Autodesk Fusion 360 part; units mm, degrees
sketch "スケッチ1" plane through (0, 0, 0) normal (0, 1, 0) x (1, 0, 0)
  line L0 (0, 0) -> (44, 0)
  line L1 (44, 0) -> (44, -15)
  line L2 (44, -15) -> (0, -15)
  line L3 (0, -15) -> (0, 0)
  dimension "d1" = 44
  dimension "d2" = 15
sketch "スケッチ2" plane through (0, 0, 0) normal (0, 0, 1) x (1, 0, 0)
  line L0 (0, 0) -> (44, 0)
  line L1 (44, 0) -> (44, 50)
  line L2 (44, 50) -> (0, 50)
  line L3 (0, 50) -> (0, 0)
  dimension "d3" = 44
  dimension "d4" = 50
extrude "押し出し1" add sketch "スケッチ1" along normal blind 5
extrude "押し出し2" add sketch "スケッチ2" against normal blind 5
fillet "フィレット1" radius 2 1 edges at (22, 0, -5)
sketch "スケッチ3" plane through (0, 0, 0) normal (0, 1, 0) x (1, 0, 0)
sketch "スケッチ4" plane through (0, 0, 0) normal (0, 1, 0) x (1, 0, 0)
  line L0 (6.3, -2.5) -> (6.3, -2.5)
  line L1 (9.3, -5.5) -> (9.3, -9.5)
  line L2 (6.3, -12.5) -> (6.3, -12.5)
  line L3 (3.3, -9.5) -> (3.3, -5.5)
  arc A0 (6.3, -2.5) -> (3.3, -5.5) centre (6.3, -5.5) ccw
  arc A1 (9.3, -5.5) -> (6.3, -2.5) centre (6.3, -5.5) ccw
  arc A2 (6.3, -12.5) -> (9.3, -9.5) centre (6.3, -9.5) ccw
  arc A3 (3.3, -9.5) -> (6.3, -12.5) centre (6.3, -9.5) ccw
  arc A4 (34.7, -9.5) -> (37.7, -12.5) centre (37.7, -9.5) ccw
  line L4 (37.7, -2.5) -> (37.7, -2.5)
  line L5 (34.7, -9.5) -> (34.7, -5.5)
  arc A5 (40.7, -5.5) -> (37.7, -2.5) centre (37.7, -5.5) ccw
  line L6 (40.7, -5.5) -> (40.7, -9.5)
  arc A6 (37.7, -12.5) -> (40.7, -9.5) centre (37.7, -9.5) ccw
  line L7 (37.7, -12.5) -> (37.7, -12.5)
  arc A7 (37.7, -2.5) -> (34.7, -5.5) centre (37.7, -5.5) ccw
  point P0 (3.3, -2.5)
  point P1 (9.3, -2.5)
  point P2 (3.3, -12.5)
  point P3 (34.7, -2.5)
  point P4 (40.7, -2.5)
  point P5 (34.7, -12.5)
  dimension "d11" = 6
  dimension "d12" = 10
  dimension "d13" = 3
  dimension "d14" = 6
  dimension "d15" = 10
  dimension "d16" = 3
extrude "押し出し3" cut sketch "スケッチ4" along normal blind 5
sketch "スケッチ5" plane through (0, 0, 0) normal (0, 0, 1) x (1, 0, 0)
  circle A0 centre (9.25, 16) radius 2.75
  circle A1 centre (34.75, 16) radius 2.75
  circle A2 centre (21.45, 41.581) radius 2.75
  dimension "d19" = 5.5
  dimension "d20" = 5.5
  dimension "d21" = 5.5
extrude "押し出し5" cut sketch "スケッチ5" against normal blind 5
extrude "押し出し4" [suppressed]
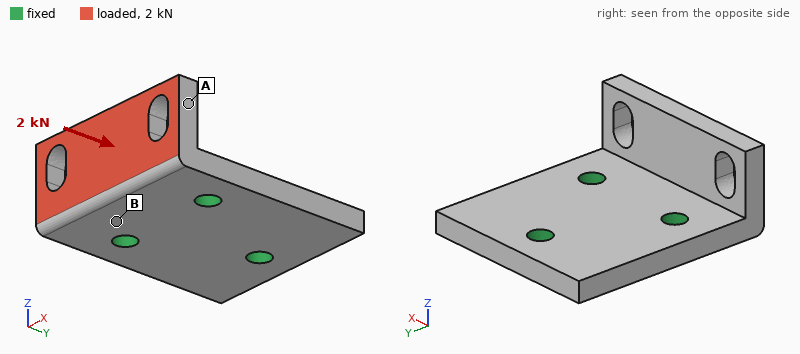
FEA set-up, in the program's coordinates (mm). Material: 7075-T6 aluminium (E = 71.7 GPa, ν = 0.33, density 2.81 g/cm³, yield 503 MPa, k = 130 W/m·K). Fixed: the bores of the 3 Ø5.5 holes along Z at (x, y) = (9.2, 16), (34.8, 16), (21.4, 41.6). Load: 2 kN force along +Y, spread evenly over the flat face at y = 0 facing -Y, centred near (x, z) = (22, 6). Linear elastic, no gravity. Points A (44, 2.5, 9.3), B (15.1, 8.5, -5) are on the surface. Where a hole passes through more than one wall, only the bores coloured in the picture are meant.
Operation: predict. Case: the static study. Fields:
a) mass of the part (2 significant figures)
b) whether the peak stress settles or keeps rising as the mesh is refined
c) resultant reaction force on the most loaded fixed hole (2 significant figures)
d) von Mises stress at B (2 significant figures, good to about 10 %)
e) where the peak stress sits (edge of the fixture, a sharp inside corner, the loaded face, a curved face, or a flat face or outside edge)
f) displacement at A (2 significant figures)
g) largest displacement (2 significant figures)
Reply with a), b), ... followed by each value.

a) 38 g
b) keeps rising
c) 930 N
d) 71 MPa
e) edge of the fixture
f) 0.094 mm
g) 0.15 mm
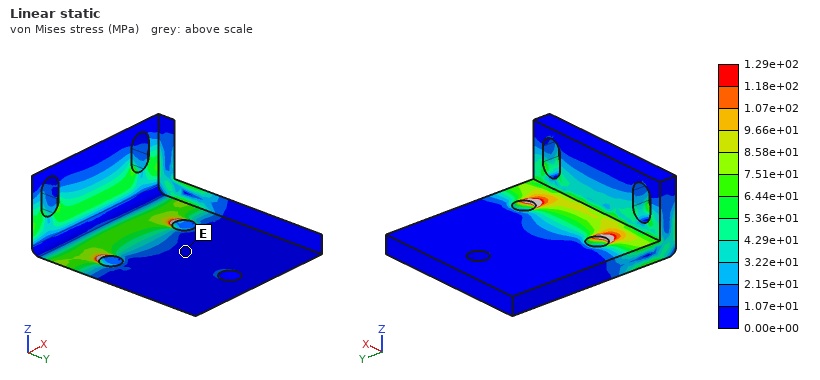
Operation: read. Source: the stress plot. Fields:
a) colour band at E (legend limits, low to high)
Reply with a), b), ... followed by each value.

a) 0.00e+00 to 1.07e+01 MPa
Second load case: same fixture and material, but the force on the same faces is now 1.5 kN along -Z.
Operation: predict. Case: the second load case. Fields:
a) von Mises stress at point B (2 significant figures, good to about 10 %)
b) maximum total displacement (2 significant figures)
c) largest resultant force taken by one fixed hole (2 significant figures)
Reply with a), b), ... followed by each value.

a) 59 MPa
b) 0.12 mm
c) 810 N
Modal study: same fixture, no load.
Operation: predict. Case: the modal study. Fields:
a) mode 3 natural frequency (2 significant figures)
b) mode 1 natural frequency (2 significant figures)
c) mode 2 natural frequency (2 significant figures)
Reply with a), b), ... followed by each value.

a) 11 kHz
b) 6300 Hz
c) 9900 Hz
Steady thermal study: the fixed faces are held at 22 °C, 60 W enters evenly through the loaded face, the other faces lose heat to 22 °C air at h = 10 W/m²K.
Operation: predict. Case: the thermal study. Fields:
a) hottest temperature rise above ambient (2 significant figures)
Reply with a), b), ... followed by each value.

a) 47 K
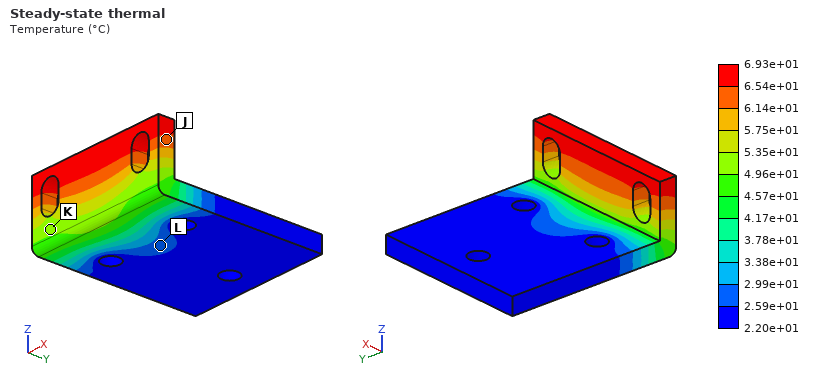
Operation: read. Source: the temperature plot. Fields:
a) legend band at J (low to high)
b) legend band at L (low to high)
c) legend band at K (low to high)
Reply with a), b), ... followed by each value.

a) 6.14e+01 to 6.54e+01 °C
b) 2.59e+01 to 2.99e+01 °C
c) 4.96e+01 to 5.35e+01 °C
